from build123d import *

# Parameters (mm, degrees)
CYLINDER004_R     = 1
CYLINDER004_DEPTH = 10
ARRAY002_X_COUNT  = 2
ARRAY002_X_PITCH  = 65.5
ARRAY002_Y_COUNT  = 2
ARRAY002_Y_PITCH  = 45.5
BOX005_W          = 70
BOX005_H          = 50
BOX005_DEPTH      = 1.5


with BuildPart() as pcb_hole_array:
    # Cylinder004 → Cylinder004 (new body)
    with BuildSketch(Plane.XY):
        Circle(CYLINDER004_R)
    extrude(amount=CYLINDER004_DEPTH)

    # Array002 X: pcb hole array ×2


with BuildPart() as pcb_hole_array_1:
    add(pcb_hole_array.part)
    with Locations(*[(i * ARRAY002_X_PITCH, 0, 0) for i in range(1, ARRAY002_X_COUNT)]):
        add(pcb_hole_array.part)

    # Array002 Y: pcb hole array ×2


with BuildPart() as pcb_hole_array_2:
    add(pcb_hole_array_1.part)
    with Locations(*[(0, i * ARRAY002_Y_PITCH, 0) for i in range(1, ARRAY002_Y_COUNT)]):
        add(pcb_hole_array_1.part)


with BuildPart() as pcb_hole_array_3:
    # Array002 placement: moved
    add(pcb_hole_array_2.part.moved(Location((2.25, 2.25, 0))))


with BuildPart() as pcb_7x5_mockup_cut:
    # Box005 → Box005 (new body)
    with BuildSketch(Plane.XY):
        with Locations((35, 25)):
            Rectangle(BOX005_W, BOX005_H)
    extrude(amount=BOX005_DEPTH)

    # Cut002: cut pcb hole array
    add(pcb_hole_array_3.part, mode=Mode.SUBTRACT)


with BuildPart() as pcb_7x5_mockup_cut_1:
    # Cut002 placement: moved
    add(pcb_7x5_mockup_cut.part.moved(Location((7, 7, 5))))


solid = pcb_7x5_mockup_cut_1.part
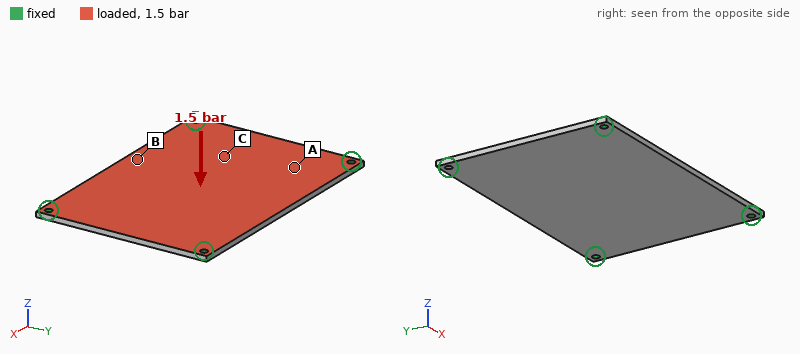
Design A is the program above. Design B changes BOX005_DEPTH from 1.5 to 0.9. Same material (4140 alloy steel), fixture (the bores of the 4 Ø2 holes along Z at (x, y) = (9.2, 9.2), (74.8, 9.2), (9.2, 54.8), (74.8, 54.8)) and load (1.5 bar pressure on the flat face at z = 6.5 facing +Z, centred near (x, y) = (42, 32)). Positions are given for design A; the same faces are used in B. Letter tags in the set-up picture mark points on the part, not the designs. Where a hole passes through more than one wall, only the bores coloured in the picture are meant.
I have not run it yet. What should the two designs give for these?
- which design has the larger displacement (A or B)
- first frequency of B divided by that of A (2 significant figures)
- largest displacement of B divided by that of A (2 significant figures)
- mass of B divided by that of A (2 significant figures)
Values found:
B
0.61
4.5
0.60
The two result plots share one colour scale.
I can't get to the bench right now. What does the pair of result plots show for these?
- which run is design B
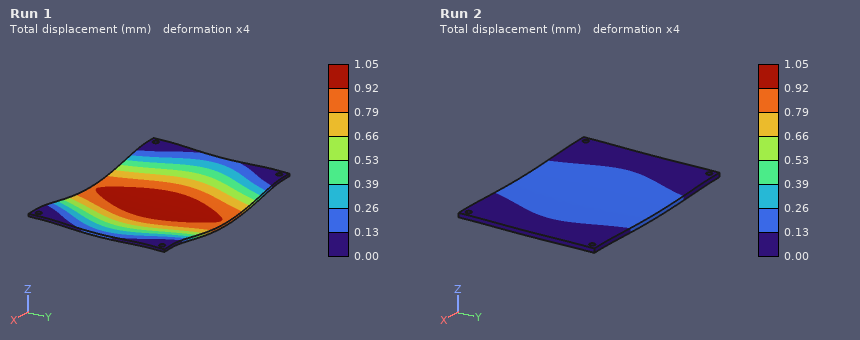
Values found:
Run 1
